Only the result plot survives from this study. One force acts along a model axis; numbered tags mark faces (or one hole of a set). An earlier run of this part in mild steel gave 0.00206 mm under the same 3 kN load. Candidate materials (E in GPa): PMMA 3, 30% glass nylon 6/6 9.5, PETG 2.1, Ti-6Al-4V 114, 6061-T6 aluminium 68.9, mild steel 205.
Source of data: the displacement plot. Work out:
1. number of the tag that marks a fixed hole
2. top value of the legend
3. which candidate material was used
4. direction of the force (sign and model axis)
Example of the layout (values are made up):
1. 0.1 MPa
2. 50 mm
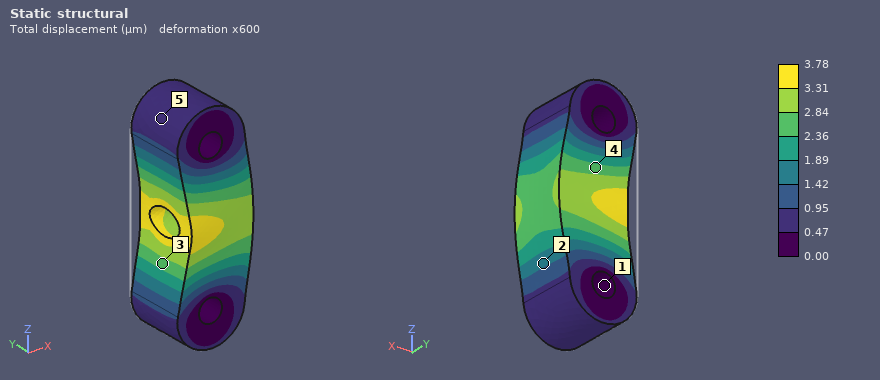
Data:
1. 1
2. 3.78 µm
3. Ti-6Al-4V
4. +X
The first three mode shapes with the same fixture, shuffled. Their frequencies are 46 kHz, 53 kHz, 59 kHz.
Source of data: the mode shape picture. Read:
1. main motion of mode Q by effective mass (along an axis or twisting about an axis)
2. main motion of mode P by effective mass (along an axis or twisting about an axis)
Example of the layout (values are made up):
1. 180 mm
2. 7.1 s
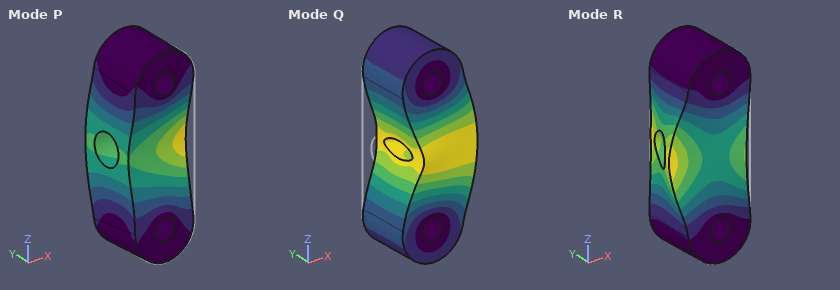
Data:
1. along X
2. along Y
